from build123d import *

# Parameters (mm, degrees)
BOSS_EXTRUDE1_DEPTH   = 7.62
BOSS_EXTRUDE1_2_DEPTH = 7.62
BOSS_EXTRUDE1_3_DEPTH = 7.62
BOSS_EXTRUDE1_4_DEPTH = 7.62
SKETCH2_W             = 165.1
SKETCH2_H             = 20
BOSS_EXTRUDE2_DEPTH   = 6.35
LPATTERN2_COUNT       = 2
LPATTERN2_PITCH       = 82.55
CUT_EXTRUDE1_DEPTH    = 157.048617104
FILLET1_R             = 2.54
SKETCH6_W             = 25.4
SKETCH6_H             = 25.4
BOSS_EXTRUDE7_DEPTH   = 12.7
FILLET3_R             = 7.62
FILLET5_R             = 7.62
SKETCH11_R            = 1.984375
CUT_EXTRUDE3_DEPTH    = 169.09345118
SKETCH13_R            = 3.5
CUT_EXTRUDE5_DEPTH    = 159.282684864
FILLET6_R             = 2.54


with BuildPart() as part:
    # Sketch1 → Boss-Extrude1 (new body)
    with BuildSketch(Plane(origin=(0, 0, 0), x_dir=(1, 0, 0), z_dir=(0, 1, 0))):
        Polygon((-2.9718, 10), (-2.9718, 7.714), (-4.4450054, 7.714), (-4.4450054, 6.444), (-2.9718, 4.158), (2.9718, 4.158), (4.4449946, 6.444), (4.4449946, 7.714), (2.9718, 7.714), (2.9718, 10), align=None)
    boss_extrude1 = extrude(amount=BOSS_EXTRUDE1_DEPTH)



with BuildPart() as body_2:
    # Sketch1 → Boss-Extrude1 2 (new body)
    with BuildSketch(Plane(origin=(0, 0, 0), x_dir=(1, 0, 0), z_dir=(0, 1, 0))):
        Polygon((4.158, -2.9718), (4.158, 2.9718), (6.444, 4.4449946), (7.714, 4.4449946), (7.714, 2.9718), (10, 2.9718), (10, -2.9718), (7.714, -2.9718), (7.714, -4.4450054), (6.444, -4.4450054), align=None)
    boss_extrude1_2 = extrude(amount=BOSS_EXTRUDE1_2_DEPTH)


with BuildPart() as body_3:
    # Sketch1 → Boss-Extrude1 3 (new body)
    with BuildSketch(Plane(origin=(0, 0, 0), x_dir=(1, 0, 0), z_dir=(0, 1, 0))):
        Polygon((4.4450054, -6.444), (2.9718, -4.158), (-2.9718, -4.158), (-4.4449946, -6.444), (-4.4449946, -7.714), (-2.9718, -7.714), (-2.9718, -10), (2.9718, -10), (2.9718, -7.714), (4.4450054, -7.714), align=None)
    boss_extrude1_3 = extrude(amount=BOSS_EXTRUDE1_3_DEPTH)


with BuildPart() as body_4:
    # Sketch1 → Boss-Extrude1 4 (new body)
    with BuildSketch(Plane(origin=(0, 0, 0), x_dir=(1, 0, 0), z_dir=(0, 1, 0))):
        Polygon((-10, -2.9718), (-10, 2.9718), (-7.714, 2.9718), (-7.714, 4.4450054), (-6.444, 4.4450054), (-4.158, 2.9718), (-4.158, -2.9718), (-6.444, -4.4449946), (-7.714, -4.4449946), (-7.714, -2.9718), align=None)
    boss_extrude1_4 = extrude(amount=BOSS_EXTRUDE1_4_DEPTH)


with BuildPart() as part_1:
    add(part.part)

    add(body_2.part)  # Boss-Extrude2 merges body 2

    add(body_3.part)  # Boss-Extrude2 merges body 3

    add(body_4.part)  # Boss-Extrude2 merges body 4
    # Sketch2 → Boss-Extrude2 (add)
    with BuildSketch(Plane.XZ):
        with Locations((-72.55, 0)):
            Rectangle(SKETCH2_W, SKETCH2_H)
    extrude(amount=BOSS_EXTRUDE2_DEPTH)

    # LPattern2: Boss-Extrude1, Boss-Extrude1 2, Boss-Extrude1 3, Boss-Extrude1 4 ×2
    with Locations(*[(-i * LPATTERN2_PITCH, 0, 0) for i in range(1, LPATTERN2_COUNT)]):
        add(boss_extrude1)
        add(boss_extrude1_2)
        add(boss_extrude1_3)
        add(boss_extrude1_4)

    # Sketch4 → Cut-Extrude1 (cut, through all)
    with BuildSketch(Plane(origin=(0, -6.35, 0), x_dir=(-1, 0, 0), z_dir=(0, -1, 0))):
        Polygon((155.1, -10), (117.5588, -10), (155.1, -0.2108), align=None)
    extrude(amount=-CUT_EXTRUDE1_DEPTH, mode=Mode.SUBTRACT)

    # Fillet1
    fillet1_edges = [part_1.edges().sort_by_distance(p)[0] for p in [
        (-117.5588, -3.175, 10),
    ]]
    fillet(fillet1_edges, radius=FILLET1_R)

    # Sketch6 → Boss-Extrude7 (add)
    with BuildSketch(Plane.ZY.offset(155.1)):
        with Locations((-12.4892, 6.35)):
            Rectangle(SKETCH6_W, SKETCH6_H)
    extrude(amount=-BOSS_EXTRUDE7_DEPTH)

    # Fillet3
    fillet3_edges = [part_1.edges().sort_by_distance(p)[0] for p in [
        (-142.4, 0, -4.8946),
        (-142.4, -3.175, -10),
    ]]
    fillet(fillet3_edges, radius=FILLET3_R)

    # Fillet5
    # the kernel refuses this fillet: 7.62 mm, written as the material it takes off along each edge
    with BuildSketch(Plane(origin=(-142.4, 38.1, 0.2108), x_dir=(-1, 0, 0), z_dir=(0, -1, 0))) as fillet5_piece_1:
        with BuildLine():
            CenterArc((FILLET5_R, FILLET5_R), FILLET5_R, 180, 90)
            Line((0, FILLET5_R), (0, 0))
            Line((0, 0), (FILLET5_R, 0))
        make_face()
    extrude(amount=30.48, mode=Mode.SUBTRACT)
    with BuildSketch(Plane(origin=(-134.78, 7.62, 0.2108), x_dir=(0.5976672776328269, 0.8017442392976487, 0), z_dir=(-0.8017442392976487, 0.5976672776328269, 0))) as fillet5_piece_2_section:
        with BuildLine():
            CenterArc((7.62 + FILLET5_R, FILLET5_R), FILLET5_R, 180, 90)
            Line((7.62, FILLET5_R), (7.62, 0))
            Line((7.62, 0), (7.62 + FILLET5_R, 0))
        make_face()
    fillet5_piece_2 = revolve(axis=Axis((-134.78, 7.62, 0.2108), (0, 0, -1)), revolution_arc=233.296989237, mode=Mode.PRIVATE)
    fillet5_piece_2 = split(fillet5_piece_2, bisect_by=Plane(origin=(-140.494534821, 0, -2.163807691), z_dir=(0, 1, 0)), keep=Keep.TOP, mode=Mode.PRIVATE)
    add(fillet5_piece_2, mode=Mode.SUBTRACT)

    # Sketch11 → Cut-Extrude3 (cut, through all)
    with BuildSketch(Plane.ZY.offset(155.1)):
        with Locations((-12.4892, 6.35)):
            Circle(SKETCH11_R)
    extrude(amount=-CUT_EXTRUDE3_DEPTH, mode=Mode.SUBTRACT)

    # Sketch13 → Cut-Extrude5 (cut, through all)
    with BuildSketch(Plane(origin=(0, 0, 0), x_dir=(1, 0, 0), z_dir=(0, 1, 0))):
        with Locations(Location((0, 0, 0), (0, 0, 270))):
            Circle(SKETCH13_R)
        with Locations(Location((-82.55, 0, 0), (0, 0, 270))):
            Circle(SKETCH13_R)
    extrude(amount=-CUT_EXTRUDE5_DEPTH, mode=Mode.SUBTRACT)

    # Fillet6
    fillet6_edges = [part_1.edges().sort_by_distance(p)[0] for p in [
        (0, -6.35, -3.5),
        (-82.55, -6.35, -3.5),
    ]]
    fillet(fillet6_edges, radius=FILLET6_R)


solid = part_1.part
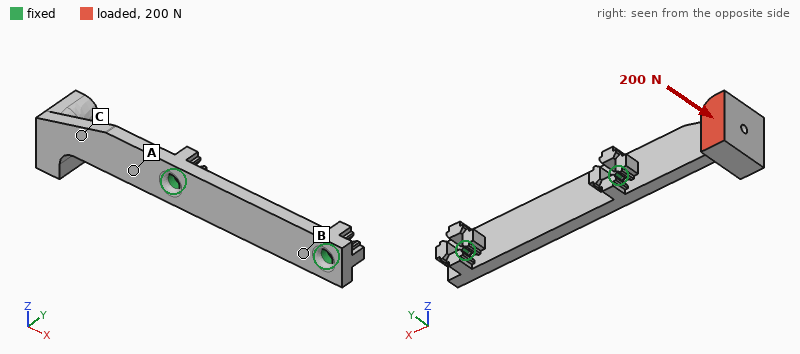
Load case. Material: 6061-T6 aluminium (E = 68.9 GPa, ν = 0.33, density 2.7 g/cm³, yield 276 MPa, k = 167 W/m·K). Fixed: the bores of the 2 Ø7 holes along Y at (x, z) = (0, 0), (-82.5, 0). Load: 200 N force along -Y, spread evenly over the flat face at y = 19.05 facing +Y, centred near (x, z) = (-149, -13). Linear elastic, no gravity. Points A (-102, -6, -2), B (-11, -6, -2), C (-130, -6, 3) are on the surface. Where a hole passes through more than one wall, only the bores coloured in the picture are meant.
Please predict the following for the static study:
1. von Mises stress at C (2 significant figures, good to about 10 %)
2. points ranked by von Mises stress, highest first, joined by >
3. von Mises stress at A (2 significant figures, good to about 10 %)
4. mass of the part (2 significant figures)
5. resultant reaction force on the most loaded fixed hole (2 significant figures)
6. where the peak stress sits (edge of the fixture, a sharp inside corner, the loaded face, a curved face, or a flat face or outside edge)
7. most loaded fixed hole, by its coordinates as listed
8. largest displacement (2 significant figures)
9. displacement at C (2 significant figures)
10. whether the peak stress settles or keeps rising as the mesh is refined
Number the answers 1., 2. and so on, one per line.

1. 38 MPa
2. A > C > B
3. 70 MPa
4. 78 g
5. 240 N
6. edge of the fixture
7. (-82.5, 0)
8. 0.95 mm
9. 0.38 mm
10. keeps rising
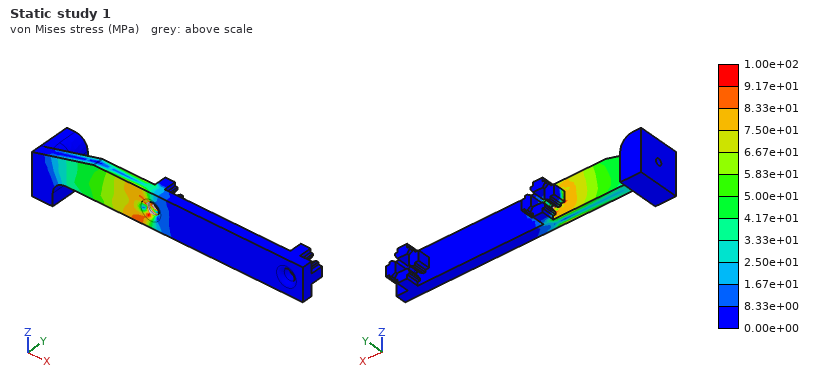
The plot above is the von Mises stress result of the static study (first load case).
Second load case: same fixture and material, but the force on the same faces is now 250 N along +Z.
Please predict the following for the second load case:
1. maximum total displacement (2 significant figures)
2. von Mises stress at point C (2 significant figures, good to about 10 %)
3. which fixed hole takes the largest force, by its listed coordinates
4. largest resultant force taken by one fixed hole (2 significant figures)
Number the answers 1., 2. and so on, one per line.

1. 0.45 mm
2. 39 MPa
3. (-82.5, 0)
4. 330 N
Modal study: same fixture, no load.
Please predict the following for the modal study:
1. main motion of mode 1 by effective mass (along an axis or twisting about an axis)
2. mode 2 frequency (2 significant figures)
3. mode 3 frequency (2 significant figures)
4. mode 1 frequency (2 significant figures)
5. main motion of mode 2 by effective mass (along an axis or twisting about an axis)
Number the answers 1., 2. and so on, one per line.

1. along Y
2. 1200 Hz
3. 2400 Hz
4. 520 Hz
5. along Z
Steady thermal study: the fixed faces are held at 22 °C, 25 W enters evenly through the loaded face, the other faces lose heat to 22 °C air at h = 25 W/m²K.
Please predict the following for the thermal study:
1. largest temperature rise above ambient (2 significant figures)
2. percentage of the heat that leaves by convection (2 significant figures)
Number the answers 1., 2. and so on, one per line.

1. 75 K
2. 24 %
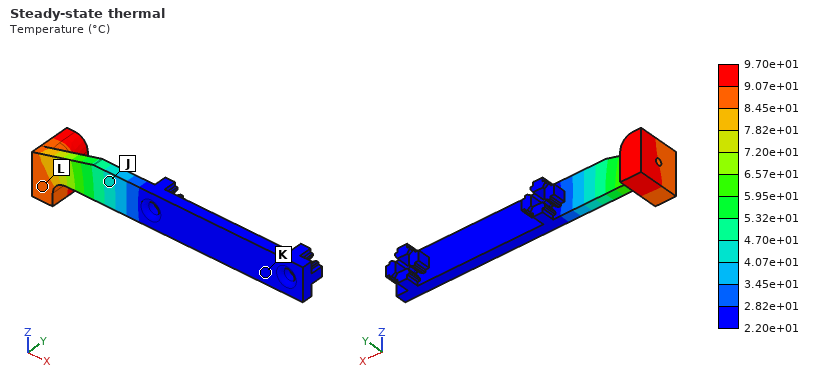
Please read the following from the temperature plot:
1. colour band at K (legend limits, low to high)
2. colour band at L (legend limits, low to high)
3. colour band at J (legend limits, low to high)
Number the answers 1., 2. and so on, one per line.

1. 2.20e+01 to 2.82e+01 °C
2. 8.45e+01 to 9.07e+01 °C
3. 4.07e+01 to 4.70e+01 °C
